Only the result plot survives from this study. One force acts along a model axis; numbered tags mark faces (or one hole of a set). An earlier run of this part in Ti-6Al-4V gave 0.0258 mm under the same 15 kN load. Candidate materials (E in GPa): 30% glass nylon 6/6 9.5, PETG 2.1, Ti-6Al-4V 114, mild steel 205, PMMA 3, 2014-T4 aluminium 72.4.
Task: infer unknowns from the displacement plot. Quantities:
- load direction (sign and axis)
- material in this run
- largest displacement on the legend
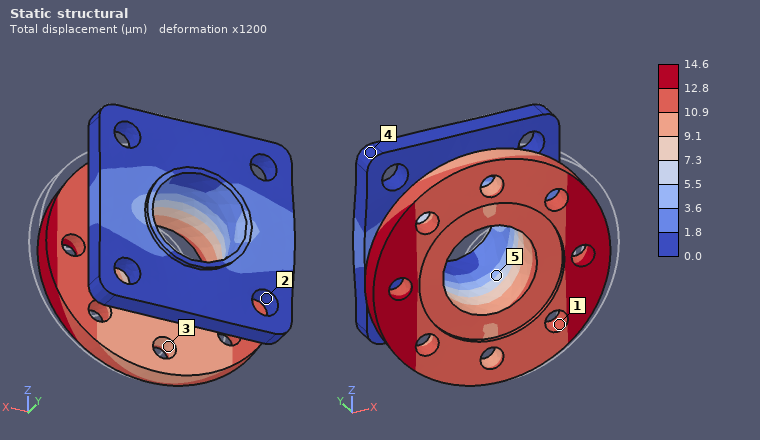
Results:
-X
mild steel
14.6 µm
